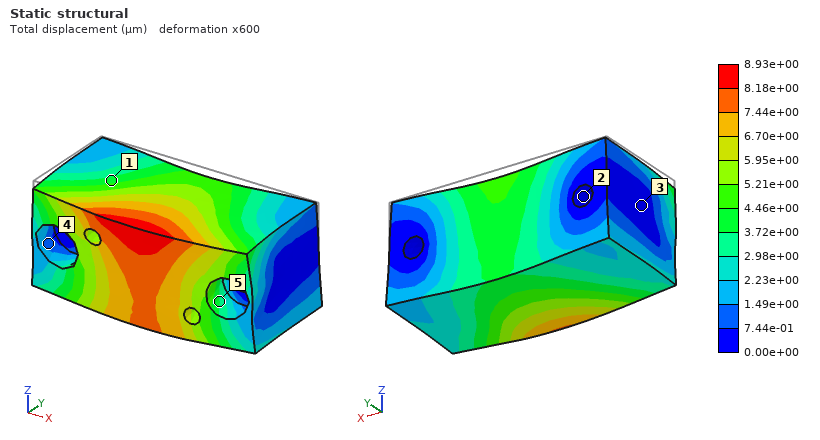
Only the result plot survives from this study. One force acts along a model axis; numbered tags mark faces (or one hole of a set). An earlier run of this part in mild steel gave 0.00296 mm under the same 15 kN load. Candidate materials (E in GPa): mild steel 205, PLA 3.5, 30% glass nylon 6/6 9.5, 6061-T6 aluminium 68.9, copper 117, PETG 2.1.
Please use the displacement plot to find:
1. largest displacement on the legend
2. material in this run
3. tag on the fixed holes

8.93e+00 µm
6061-T6 aluminium
2
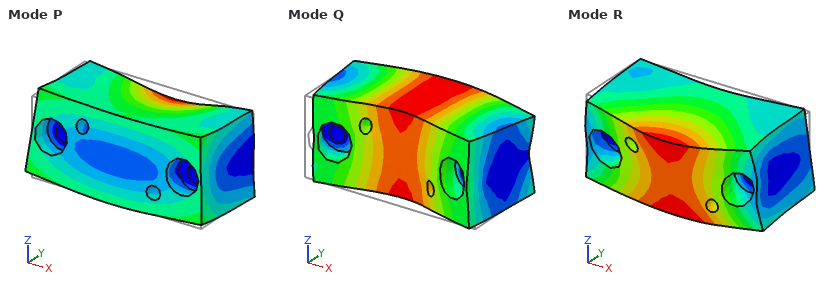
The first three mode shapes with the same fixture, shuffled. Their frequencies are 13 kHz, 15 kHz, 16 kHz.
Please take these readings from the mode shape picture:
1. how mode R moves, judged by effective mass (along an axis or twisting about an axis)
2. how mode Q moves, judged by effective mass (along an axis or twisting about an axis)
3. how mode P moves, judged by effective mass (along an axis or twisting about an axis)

along Z
along Y
along Z
